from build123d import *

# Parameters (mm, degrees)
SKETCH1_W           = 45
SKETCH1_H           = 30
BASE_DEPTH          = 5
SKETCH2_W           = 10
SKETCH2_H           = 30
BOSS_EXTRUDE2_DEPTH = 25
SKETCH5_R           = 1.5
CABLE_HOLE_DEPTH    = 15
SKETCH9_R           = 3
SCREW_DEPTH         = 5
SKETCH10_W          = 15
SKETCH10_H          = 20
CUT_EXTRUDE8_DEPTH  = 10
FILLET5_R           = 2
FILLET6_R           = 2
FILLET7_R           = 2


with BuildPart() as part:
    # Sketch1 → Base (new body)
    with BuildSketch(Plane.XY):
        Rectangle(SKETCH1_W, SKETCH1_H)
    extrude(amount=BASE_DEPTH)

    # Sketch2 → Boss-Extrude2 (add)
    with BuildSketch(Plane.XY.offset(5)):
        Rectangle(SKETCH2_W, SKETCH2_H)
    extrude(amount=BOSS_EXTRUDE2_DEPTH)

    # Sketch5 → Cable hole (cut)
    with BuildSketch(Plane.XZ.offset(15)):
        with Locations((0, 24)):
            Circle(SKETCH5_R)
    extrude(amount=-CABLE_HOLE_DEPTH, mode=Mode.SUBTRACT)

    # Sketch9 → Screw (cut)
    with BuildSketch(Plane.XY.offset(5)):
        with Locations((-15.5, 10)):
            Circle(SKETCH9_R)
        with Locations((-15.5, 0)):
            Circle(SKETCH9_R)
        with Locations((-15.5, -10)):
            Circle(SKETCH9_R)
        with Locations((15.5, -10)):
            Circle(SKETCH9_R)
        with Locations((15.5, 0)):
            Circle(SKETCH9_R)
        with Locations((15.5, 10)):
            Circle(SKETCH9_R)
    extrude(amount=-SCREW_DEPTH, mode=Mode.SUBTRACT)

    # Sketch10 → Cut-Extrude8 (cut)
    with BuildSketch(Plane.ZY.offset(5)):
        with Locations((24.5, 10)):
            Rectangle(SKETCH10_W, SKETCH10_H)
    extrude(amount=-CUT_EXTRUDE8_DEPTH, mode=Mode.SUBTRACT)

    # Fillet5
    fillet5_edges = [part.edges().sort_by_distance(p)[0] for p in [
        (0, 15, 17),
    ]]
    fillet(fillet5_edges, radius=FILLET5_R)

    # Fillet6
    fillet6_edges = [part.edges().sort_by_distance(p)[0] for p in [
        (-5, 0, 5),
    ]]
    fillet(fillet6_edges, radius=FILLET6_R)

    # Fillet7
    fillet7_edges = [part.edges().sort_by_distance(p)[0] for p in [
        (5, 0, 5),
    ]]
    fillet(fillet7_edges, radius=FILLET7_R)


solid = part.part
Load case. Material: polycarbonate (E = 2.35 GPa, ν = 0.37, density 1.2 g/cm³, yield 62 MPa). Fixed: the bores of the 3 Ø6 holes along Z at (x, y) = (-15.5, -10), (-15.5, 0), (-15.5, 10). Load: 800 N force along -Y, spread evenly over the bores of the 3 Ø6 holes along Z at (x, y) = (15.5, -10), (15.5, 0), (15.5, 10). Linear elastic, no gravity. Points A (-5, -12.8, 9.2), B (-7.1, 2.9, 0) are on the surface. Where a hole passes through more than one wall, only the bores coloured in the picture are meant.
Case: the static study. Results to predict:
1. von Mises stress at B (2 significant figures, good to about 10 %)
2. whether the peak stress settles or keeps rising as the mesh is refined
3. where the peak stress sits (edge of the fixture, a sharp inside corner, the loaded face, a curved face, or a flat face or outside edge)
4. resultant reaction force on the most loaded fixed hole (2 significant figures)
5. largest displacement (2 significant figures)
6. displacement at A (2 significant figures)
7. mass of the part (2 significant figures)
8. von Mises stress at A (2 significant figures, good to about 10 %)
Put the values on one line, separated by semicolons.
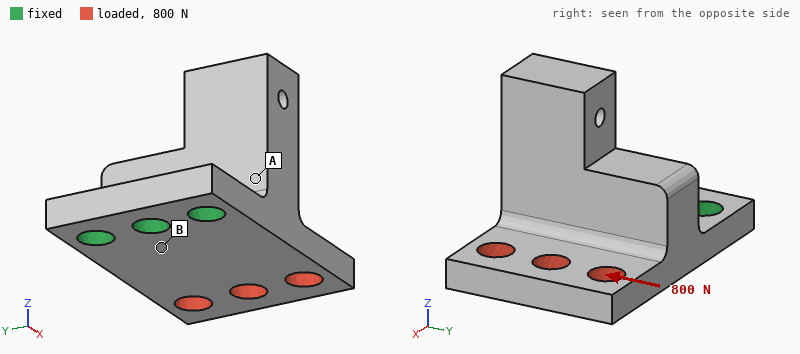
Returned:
15 MPa; keeps rising; edge of the fixture; 1.1 kN; 0.64 mm; 0.16 mm; 14 g; 4.4 MPa
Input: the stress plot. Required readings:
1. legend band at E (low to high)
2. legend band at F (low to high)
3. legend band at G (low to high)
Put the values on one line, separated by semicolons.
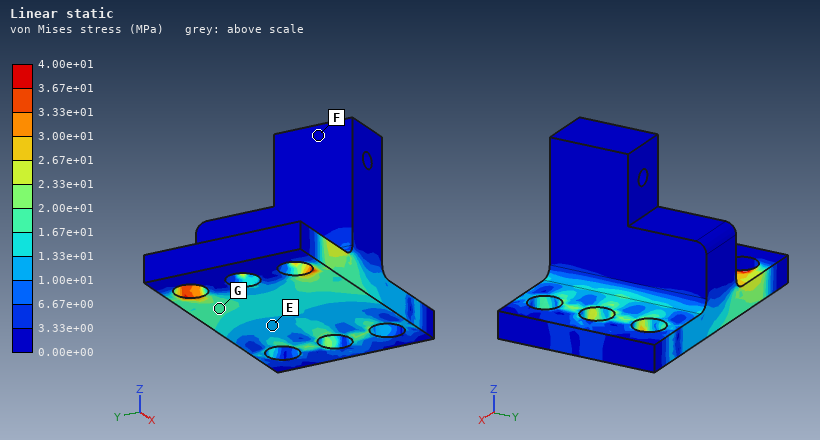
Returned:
1.00e+01 to 1.33e+01 MPa; 0.00e+00 to 3.33e+00 MPa; 1.67e+01 to 2.00e+01 MPa
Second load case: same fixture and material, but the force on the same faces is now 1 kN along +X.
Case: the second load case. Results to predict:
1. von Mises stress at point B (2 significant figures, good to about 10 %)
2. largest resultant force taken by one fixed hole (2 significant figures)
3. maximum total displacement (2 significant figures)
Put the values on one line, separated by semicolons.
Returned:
6.6 MPa; 350 N; 0.15 mm
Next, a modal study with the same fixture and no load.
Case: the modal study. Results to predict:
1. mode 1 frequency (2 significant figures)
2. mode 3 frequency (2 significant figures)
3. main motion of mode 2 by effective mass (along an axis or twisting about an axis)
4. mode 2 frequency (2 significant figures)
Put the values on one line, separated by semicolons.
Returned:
760 Hz; 3100 Hz; along Y; 1900 Hz
